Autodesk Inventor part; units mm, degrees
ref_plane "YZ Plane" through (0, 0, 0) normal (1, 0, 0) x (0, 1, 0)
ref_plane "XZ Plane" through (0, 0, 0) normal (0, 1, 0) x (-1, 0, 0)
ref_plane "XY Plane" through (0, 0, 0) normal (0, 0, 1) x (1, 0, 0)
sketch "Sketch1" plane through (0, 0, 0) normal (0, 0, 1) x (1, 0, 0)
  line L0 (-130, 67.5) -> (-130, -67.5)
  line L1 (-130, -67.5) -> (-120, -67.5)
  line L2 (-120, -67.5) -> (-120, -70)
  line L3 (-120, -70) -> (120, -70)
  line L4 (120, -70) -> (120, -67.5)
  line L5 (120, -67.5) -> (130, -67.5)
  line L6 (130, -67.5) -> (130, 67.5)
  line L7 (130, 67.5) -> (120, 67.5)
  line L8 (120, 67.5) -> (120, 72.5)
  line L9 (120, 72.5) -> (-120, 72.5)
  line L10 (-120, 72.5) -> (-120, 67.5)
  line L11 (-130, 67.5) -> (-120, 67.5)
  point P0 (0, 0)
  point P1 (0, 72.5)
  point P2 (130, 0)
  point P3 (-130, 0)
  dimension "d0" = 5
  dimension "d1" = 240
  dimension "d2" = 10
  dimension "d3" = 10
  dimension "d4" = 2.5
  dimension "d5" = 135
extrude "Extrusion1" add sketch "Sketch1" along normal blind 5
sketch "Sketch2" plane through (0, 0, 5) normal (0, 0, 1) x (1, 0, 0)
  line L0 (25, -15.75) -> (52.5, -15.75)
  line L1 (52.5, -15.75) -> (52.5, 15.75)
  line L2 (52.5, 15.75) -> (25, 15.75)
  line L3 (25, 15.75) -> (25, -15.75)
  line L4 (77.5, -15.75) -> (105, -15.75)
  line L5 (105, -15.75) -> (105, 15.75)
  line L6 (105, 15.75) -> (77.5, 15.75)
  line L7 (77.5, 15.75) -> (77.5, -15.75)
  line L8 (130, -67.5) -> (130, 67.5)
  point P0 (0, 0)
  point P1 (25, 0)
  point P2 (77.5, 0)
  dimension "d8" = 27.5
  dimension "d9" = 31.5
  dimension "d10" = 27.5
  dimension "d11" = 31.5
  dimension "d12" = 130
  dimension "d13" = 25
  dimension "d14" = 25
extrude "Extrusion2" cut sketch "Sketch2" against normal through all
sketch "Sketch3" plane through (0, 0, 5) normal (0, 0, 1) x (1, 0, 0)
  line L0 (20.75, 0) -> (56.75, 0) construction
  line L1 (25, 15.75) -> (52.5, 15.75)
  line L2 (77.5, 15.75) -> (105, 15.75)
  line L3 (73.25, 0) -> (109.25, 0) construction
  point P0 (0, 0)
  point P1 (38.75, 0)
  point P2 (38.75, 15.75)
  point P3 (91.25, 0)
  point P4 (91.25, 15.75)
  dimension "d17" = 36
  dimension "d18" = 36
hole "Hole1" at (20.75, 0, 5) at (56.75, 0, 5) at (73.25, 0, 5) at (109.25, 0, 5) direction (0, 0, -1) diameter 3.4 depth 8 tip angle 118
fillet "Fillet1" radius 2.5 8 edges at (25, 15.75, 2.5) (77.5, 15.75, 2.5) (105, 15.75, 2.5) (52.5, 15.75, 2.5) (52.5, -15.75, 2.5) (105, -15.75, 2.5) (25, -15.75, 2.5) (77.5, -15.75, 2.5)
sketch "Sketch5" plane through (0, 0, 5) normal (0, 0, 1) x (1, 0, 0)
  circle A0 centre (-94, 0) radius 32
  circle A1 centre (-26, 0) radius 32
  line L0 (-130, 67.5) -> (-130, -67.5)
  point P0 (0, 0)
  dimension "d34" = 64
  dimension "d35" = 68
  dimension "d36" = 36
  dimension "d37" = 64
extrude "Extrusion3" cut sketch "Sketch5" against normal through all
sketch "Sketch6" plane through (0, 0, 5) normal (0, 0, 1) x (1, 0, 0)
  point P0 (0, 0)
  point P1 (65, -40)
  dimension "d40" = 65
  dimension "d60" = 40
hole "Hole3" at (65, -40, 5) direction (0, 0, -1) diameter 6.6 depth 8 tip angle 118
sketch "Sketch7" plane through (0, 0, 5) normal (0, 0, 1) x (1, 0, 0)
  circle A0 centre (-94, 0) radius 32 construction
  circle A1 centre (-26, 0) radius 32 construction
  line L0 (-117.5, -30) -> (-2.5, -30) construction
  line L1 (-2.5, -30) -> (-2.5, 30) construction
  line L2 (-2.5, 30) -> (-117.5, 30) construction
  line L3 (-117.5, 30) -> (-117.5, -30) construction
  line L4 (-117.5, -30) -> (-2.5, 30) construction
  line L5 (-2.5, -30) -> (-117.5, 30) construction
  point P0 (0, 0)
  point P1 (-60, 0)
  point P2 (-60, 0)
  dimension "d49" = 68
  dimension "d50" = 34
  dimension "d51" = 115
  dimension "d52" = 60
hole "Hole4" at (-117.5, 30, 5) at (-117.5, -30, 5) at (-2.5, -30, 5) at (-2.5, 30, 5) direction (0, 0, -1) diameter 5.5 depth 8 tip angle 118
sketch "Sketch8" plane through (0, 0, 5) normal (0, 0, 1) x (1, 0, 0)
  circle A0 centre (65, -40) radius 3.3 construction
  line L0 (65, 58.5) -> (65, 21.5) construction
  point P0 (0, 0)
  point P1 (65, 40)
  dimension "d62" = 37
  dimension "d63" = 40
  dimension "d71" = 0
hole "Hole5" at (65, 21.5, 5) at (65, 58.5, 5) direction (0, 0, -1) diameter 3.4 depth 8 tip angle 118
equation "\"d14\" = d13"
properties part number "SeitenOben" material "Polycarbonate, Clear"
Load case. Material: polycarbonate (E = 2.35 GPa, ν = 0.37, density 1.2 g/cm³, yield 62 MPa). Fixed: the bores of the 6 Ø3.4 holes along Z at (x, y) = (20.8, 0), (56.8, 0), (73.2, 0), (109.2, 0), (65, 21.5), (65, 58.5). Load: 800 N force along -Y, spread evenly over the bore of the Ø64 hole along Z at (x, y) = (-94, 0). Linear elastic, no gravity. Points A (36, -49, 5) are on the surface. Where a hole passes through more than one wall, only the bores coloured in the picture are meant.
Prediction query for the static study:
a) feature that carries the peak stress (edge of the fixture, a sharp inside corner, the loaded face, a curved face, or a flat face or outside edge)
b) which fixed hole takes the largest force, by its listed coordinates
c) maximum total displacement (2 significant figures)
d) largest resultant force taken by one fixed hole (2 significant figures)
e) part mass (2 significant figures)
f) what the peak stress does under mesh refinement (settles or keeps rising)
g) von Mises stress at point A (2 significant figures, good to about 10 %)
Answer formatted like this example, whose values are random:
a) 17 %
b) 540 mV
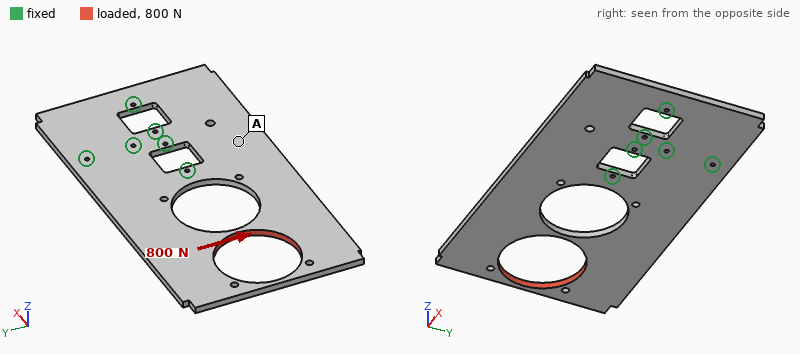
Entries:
a) edge of the fixture
b) (20.8, 0)
c) 3.1 mm
d) 1.4 kN
e) 170 g
f) keeps rising
g) 4.3 MPa
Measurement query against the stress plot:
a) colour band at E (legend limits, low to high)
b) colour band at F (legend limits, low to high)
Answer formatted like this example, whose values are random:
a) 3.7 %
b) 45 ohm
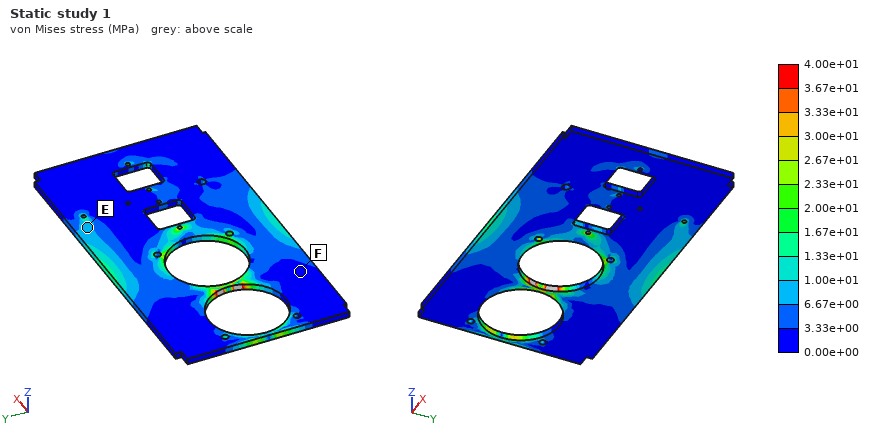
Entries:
a) 6.67e+00 to 1.00e+01 MPa
b) 0.00e+00 to 3.33e+00 MPa
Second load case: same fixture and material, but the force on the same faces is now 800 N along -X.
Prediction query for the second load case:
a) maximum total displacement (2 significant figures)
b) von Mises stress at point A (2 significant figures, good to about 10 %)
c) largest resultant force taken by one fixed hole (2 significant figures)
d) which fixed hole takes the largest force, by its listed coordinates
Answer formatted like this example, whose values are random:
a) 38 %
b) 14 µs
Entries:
a) 0.45 mm
b) 1.6 MPa
c) 200 N
d) (20.8, 0)
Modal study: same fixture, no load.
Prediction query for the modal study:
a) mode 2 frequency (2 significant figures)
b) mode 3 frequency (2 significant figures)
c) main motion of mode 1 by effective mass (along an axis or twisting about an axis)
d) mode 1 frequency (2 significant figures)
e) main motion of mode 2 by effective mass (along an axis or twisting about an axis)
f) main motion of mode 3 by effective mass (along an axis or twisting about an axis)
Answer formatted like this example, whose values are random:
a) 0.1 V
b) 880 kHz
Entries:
a) 75 Hz
b) 170 Hz
c) along Z
d) 40 Hz
e) twisting about X
f) along Z
